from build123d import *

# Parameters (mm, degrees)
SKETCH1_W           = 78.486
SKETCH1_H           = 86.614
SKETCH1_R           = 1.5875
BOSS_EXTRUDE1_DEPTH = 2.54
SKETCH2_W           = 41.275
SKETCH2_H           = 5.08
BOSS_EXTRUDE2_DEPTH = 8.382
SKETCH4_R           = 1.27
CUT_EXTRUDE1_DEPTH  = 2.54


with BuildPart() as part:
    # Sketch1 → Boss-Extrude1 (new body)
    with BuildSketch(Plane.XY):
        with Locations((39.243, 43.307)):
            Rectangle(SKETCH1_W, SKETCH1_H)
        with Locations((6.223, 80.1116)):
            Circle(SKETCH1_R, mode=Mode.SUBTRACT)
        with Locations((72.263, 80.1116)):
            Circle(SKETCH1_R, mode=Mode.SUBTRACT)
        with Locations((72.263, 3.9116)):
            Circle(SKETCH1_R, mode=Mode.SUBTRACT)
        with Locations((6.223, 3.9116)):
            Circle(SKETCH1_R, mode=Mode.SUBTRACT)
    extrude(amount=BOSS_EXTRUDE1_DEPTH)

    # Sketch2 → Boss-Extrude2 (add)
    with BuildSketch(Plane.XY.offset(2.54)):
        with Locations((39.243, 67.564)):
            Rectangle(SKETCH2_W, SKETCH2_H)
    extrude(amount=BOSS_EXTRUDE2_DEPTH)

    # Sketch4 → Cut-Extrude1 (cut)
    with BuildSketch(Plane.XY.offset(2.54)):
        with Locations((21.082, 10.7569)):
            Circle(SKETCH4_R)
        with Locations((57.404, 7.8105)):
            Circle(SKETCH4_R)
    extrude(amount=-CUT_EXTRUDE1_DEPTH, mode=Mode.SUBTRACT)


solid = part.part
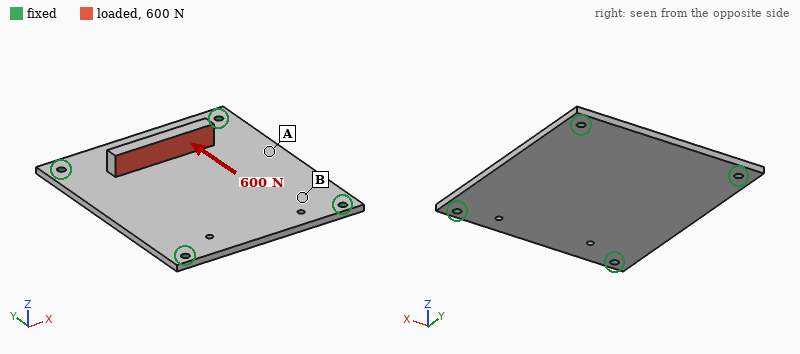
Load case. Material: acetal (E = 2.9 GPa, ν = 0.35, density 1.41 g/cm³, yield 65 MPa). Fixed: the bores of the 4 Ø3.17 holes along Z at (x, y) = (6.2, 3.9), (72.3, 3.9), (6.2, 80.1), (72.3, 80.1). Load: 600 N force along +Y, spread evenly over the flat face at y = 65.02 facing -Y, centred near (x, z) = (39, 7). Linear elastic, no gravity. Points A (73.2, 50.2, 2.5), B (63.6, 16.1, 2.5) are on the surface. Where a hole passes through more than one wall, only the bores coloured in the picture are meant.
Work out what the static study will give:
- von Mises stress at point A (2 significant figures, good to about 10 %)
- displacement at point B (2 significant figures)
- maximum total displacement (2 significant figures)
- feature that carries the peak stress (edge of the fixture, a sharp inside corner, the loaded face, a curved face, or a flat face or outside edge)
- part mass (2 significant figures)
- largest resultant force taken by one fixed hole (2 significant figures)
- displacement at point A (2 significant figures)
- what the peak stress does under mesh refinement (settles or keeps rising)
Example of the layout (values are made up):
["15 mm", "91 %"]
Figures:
["10.0 MPa", "0.37 mm", "1.4 mm", "edge of the fixture", "27 g", "200 N", "0.95 mm", "keeps rising"]
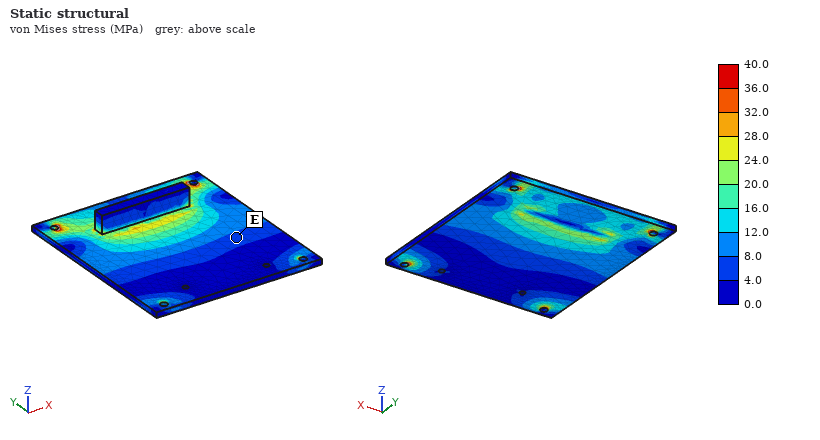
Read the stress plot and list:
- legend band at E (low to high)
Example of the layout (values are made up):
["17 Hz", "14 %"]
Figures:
["4.0 to 8.0 MPa"]
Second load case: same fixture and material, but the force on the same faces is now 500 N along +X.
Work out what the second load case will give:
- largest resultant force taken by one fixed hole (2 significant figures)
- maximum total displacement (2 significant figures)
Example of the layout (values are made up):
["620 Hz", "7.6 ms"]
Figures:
["210 N", "0.30 mm"]
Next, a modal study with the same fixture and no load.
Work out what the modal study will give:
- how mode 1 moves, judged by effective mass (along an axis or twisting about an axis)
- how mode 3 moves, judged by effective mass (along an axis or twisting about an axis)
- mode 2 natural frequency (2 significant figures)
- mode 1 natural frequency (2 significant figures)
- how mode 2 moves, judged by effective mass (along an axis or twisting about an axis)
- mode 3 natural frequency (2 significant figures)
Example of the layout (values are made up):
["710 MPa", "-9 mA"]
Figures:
["along Z", "twisting about X", "780 Hz", "480 Hz", "twisting about Y", "890 Hz"]
